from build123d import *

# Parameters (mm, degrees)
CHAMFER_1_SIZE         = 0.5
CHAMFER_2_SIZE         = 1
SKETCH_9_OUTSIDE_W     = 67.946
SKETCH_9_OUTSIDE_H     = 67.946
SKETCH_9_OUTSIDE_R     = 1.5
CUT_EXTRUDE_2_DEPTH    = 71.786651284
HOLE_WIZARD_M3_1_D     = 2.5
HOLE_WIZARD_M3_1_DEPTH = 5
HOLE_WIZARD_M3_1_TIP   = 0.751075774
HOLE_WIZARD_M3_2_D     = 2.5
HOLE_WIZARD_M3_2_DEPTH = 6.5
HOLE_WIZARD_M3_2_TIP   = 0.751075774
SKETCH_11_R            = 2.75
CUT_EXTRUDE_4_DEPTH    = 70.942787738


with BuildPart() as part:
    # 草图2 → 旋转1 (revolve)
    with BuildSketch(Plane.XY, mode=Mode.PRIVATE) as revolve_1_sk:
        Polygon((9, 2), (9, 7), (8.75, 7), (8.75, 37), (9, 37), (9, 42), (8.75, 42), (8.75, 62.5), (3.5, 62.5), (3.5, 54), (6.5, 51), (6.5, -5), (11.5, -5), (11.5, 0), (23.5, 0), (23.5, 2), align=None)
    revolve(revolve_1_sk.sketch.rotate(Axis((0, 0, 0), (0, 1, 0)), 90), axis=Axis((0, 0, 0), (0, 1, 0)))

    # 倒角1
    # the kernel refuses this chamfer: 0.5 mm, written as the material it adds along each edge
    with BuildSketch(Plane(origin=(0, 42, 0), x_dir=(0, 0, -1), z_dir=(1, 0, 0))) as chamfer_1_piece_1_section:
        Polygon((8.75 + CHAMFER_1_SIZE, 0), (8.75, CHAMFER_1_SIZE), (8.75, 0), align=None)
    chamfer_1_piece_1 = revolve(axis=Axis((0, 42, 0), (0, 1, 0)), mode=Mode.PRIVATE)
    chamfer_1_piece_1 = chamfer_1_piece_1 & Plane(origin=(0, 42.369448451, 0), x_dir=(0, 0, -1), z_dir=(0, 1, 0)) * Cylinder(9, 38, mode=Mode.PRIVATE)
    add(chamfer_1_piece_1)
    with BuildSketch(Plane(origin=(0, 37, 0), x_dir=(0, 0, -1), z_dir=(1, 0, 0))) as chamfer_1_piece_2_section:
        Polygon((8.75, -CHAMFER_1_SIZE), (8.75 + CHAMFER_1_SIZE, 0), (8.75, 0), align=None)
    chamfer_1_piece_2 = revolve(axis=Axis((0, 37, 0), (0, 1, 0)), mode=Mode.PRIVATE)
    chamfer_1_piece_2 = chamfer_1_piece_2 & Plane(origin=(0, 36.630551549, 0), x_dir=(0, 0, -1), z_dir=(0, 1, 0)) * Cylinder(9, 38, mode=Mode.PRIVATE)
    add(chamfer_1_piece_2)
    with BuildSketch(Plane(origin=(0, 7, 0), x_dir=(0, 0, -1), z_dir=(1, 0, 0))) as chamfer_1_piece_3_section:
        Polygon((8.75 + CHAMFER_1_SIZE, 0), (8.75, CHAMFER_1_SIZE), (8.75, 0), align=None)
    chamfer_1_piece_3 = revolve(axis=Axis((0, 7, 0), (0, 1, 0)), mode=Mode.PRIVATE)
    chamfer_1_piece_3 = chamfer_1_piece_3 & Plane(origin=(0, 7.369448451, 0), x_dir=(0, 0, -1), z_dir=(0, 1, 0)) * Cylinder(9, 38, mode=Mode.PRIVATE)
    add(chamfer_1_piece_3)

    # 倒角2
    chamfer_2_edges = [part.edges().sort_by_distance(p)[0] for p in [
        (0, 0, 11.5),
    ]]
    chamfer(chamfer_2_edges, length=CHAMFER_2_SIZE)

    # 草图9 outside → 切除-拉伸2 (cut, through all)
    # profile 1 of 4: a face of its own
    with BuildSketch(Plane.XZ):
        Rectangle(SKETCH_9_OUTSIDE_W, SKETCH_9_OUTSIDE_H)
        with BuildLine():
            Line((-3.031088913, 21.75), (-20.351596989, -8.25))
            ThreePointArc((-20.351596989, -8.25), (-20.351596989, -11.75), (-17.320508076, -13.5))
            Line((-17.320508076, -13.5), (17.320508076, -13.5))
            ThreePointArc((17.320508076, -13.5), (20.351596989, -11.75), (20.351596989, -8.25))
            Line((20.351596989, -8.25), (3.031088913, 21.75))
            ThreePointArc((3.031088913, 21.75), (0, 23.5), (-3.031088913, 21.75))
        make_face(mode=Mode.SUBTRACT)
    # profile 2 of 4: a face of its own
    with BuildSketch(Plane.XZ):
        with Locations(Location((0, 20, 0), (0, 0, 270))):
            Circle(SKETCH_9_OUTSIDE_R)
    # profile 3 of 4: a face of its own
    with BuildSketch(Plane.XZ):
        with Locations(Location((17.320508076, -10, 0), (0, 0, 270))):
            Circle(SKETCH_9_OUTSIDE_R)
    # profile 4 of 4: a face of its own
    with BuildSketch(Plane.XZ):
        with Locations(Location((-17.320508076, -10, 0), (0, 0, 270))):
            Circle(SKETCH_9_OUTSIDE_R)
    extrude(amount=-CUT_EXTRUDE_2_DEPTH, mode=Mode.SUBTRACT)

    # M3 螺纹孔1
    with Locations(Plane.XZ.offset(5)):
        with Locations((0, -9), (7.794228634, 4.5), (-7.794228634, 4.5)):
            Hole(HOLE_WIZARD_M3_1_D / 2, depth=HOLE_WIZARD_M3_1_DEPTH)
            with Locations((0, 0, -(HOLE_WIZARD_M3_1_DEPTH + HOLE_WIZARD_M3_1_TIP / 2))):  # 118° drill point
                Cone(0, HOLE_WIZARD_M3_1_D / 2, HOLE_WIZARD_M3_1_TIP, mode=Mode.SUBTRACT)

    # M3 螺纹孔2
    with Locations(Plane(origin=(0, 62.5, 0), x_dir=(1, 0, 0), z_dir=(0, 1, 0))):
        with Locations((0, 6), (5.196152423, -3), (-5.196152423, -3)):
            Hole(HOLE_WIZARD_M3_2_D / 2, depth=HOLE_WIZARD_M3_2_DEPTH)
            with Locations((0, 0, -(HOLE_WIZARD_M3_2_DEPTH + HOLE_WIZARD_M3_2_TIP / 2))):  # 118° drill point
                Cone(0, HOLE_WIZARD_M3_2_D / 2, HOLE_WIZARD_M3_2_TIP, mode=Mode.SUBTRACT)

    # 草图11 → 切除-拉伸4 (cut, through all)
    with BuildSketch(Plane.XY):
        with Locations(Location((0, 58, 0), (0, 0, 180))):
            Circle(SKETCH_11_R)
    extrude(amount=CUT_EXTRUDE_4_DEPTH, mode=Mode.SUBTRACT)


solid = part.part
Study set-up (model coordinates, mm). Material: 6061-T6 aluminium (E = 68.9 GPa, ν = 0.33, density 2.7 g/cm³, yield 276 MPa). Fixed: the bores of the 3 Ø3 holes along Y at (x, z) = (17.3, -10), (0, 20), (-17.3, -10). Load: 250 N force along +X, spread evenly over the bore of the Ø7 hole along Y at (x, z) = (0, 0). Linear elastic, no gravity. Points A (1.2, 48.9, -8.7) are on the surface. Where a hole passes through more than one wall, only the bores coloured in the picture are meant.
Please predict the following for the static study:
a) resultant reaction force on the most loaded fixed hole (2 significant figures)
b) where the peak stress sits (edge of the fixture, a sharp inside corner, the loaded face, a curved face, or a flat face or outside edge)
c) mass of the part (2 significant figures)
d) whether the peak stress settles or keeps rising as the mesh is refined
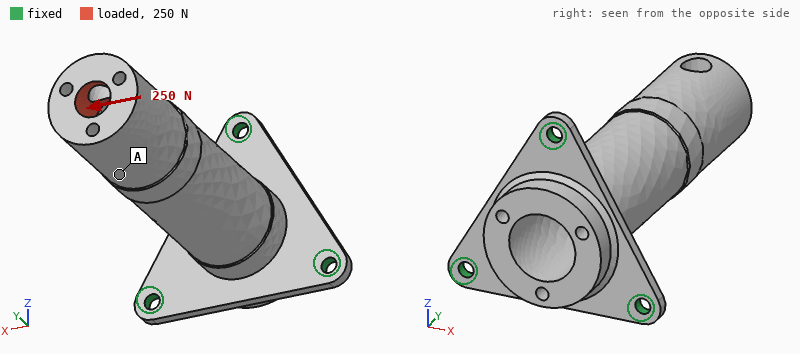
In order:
490 N
edge of the fixture
28 g
keeps rising
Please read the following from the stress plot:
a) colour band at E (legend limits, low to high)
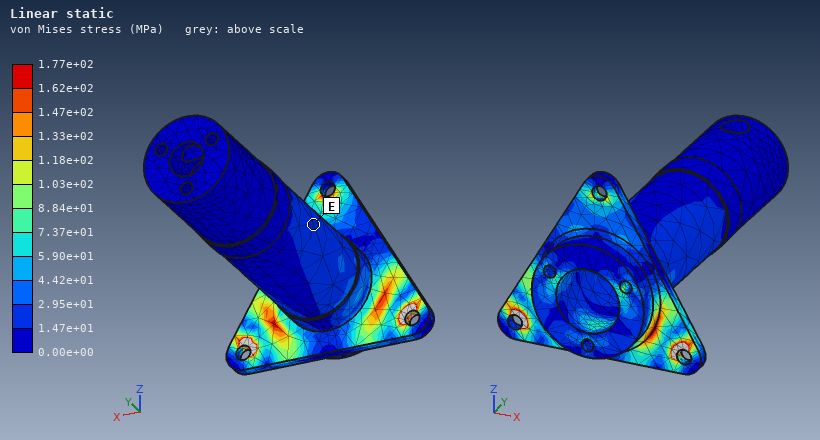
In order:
1.47e+01 to 2.95e+01 MPa
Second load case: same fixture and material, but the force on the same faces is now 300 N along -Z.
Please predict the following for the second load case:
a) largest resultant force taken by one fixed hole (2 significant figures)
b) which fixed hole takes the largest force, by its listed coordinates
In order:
670 N
(0, 20)
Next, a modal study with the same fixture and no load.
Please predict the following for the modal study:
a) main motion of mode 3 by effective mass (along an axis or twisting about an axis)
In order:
along Y
